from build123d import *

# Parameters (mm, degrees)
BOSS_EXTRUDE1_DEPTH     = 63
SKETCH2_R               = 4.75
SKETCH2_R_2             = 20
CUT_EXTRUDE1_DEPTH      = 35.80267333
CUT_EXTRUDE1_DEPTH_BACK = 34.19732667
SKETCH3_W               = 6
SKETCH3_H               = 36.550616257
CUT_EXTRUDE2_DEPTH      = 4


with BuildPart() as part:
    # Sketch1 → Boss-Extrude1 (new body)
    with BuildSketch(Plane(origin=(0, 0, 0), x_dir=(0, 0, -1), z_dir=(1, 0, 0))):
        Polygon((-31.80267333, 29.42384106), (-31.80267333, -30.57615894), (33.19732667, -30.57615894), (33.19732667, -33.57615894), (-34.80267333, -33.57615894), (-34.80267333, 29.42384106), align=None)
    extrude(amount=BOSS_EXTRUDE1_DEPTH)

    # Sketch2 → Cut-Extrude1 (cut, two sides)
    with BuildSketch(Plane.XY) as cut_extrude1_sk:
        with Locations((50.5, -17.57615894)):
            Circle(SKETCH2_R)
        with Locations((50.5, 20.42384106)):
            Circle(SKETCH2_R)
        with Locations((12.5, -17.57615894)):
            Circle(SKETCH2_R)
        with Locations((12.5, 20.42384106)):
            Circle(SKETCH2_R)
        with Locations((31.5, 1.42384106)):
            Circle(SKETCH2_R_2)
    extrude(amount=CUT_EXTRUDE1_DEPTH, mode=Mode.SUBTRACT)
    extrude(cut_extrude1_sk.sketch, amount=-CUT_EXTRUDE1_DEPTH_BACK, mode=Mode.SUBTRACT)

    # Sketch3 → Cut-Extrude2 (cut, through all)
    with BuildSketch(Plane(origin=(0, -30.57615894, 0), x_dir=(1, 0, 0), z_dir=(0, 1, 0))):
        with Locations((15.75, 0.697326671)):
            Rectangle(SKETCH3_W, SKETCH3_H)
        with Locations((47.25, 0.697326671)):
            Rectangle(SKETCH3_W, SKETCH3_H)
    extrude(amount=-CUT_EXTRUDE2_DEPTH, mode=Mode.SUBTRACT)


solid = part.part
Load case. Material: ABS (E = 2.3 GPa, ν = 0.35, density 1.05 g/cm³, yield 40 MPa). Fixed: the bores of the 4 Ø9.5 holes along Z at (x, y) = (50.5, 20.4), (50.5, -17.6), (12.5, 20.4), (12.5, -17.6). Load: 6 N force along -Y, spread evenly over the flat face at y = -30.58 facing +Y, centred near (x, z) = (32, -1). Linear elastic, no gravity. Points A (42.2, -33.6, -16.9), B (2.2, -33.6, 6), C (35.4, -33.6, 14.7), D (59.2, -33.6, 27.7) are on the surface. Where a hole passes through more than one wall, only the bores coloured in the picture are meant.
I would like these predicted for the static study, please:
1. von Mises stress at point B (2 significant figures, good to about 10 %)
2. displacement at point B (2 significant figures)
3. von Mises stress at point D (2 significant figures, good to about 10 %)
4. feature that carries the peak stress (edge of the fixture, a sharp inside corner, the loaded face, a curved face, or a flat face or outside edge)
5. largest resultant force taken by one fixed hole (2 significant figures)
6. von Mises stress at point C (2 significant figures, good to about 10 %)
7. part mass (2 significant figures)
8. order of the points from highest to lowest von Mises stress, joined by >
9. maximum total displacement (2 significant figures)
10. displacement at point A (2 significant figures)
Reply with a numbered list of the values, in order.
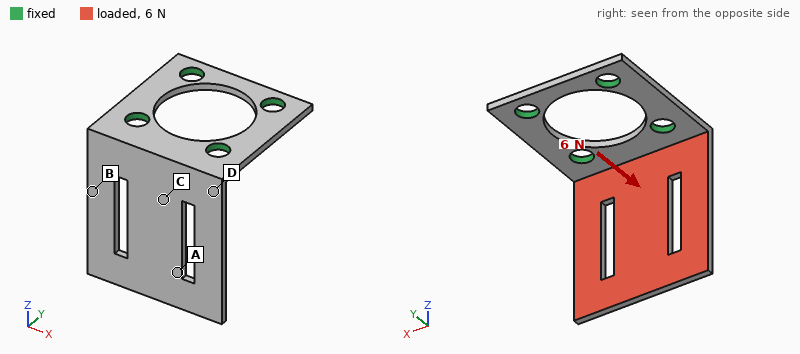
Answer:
1. 0.98 MPa
2. 0.35 mm
3. 1.7 MPa
4. a flat face or outside edge
5. 3.3 N
6. 1.2 MPa
7. 19 g
8. D > C > B > A
9. 1.2 mm
10. 0.81 mm
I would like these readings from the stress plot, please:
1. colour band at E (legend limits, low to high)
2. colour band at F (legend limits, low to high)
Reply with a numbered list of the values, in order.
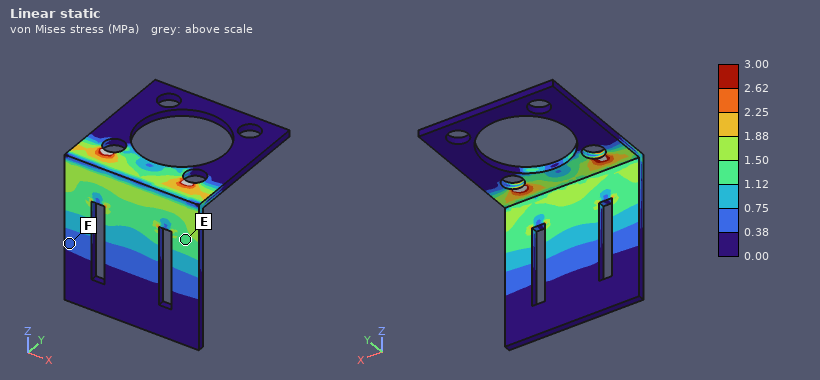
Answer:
1. 1.12 to 1.50 MPa
2. 0.38 to 0.75 MPa
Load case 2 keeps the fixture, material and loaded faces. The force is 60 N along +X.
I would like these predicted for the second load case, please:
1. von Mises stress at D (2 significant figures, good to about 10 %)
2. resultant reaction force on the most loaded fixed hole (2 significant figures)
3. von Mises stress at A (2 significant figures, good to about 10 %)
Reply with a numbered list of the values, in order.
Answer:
1. 2.5 MPa
2. 59 N
3. 0.76 MPa
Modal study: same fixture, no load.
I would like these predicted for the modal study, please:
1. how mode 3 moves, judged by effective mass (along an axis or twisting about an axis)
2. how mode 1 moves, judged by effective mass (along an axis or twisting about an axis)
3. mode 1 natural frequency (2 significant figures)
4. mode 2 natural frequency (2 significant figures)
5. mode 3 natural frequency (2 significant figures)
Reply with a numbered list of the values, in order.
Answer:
1. along X
2. along Y
3. 130 Hz
4. 350 Hz
5. 620 Hz
